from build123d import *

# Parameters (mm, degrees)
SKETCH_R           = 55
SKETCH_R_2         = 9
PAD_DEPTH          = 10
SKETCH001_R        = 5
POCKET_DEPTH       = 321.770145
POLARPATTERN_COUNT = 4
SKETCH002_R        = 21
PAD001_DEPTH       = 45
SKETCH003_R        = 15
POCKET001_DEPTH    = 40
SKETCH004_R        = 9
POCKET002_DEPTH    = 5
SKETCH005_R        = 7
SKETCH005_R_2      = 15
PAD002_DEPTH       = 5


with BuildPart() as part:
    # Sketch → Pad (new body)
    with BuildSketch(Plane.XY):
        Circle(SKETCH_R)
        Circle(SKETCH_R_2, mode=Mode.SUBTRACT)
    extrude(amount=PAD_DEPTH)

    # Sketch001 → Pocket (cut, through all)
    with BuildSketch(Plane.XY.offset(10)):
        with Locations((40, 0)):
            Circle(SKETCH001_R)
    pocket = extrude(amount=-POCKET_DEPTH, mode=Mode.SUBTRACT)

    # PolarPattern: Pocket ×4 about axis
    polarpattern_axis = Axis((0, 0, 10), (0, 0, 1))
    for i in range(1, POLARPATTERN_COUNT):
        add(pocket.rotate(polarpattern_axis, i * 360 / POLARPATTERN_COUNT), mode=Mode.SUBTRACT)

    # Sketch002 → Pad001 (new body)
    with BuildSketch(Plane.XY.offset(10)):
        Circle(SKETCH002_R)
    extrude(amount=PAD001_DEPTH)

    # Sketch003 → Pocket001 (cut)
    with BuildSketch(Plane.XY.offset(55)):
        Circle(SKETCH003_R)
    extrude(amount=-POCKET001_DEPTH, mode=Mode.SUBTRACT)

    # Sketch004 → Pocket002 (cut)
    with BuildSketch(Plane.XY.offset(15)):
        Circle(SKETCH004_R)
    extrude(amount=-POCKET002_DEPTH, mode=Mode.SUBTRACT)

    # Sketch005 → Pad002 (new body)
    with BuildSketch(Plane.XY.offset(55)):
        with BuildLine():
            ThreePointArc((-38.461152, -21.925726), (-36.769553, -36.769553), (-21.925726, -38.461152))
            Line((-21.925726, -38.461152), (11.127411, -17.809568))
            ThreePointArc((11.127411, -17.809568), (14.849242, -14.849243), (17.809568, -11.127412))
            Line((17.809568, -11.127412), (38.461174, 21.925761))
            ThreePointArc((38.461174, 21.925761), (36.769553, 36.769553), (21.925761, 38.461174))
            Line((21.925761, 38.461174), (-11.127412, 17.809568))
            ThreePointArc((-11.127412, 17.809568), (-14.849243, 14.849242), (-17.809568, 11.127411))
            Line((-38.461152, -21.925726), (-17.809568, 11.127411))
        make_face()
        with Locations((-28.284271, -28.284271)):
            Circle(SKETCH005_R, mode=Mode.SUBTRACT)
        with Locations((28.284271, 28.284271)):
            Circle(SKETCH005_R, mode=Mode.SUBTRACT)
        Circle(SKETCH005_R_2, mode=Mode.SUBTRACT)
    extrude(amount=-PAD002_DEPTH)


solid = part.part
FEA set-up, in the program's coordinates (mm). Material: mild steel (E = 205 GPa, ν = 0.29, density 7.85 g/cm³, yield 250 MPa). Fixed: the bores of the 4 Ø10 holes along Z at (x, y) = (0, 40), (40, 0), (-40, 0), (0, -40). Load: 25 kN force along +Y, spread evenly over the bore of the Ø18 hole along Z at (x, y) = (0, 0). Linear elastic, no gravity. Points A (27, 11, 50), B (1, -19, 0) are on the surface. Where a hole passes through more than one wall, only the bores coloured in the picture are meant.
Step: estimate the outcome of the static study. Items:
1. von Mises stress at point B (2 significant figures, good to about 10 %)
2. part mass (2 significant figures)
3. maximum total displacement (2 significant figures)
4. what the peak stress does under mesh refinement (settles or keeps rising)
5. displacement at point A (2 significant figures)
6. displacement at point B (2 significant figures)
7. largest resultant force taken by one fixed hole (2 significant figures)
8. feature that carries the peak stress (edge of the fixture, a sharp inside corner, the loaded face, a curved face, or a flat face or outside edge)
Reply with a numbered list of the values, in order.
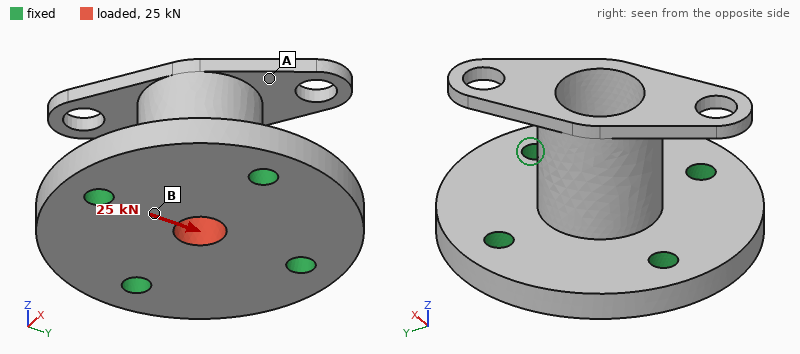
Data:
1. 30 MPa
2. 1.0 kg
3. 6.0 µm
4. keeps rising
5. 5.6 µm
6. 3.2 µm
7. 8.2 kN
8. edge of the fixture
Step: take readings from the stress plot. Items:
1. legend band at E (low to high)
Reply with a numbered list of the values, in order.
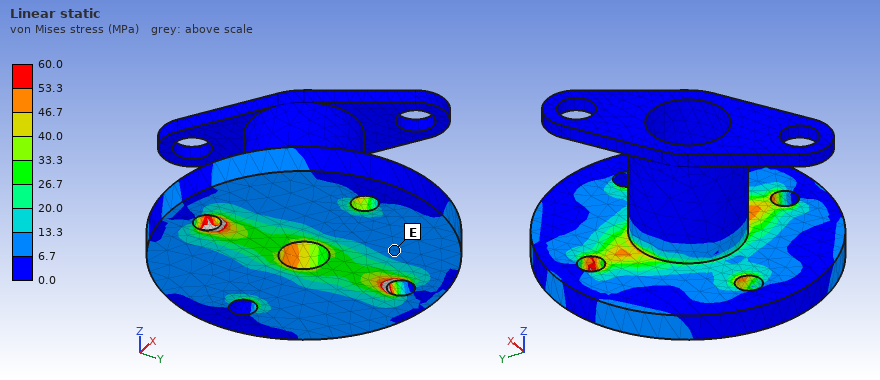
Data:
1. 6.7 to 13.3 MPa
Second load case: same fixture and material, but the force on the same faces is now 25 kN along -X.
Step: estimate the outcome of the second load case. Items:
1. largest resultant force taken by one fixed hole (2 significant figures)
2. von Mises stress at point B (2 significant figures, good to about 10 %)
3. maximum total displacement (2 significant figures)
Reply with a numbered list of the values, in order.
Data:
1. 8.2 kN
2. 9.8 MPa
3. 6.0 µm
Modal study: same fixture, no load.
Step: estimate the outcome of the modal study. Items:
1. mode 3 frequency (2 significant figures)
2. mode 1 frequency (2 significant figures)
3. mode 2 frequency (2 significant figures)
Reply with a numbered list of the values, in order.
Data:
1. 5200 Hz
2. 4100 Hz
3. 4500 Hz
